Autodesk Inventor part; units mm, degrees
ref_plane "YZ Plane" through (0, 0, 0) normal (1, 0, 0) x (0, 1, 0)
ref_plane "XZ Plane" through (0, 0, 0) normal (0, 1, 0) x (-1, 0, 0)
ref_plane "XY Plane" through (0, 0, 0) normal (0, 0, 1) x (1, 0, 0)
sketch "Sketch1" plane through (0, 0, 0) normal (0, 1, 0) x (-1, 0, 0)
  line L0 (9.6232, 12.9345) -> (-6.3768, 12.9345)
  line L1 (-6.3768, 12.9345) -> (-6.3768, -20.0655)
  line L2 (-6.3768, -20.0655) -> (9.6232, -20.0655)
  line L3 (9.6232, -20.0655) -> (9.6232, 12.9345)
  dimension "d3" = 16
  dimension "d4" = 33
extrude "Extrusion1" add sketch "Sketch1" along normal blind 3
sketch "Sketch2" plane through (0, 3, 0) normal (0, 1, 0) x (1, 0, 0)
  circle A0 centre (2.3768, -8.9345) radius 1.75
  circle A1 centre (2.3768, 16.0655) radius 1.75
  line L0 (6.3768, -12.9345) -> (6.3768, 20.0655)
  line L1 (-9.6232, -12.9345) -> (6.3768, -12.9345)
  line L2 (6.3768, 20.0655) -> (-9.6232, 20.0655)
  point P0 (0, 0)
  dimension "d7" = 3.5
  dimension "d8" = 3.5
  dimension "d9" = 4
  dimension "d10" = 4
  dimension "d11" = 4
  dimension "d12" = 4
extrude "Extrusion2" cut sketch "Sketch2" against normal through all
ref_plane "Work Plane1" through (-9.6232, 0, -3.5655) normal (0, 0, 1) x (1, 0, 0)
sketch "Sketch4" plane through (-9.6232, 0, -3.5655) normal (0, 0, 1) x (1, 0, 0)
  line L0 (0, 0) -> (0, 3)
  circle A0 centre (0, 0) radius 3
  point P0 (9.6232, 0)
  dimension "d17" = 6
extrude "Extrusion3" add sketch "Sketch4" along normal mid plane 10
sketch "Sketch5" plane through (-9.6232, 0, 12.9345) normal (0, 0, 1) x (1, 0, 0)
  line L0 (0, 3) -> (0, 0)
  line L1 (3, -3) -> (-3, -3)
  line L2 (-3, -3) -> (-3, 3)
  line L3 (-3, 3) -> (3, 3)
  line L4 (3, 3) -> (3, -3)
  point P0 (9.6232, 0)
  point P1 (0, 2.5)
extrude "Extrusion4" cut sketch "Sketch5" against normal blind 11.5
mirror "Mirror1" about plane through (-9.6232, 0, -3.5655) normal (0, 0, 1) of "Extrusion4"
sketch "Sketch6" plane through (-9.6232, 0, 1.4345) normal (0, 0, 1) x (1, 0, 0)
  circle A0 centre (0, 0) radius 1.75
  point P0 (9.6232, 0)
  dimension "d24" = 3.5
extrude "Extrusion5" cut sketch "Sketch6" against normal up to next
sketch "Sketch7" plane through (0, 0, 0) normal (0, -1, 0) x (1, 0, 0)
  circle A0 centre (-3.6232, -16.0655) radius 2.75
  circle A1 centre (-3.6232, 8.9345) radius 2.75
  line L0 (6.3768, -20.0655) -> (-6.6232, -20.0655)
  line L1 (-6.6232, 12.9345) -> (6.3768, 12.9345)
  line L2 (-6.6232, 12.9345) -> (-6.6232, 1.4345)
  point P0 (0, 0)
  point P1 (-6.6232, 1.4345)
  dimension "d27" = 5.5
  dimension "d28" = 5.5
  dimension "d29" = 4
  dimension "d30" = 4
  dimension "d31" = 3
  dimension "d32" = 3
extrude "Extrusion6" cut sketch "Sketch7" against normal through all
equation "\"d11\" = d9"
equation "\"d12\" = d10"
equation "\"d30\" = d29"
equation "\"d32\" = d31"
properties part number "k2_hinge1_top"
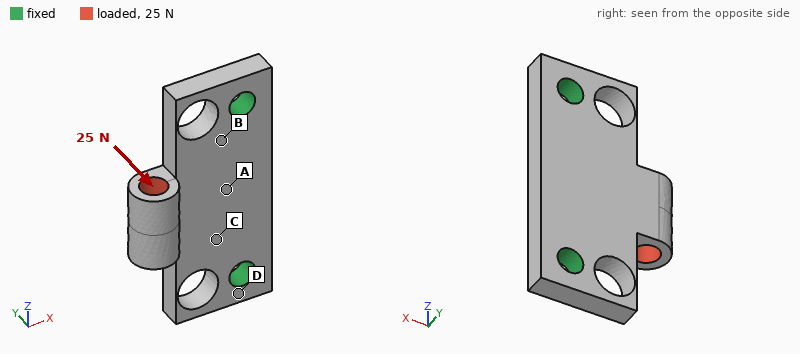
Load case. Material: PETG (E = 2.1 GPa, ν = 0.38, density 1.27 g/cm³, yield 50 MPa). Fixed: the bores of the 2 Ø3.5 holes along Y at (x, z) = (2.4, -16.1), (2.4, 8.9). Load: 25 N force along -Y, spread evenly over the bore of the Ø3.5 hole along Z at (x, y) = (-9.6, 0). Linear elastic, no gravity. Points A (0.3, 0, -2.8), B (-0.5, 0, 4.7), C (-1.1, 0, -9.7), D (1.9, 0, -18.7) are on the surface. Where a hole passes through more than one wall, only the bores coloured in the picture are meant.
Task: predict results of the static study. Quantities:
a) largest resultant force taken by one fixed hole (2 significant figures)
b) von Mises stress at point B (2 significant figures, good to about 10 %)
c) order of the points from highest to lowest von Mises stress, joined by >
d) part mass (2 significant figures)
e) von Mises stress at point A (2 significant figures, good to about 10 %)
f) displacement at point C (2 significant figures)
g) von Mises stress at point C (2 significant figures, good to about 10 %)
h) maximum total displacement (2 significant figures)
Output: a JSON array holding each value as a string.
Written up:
["13 N", "8.5 MPa", "B > C > A > D", "1.6 g", "4.4 MPa", "0.062 mm", "6.7 MPa", "0.41 mm"]
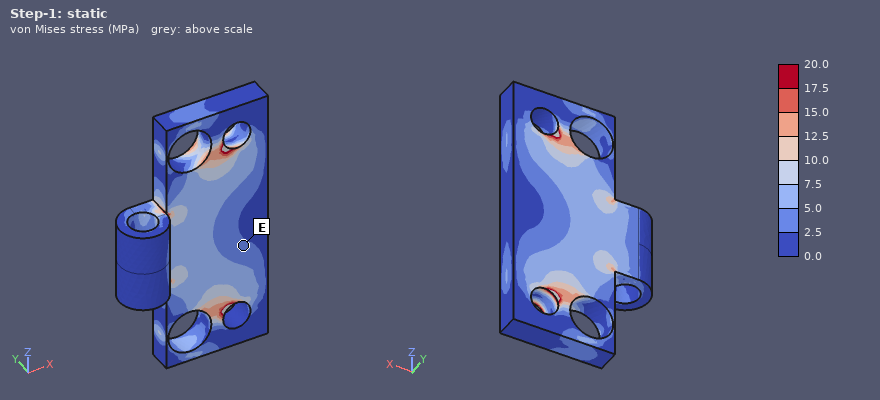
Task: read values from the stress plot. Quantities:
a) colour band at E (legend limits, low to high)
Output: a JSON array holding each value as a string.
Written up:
["2.5 to 5.0 MPa"]
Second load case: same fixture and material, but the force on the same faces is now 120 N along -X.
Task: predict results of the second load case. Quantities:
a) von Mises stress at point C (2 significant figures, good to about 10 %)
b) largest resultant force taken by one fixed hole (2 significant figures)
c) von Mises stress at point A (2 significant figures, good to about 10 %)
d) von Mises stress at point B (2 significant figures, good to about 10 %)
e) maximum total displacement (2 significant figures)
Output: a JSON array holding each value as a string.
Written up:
["8.5 MPa", "68 N", "4.7 MPa", "9.5 MPa", "0.38 mm"]
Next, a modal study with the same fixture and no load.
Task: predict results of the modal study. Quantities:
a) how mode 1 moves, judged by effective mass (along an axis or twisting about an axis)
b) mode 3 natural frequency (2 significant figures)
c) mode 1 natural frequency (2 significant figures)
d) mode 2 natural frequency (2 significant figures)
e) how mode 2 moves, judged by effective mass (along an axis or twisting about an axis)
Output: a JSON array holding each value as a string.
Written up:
["along Y", "7700 Hz", "2400 Hz", "6800 Hz", "along Y"]
